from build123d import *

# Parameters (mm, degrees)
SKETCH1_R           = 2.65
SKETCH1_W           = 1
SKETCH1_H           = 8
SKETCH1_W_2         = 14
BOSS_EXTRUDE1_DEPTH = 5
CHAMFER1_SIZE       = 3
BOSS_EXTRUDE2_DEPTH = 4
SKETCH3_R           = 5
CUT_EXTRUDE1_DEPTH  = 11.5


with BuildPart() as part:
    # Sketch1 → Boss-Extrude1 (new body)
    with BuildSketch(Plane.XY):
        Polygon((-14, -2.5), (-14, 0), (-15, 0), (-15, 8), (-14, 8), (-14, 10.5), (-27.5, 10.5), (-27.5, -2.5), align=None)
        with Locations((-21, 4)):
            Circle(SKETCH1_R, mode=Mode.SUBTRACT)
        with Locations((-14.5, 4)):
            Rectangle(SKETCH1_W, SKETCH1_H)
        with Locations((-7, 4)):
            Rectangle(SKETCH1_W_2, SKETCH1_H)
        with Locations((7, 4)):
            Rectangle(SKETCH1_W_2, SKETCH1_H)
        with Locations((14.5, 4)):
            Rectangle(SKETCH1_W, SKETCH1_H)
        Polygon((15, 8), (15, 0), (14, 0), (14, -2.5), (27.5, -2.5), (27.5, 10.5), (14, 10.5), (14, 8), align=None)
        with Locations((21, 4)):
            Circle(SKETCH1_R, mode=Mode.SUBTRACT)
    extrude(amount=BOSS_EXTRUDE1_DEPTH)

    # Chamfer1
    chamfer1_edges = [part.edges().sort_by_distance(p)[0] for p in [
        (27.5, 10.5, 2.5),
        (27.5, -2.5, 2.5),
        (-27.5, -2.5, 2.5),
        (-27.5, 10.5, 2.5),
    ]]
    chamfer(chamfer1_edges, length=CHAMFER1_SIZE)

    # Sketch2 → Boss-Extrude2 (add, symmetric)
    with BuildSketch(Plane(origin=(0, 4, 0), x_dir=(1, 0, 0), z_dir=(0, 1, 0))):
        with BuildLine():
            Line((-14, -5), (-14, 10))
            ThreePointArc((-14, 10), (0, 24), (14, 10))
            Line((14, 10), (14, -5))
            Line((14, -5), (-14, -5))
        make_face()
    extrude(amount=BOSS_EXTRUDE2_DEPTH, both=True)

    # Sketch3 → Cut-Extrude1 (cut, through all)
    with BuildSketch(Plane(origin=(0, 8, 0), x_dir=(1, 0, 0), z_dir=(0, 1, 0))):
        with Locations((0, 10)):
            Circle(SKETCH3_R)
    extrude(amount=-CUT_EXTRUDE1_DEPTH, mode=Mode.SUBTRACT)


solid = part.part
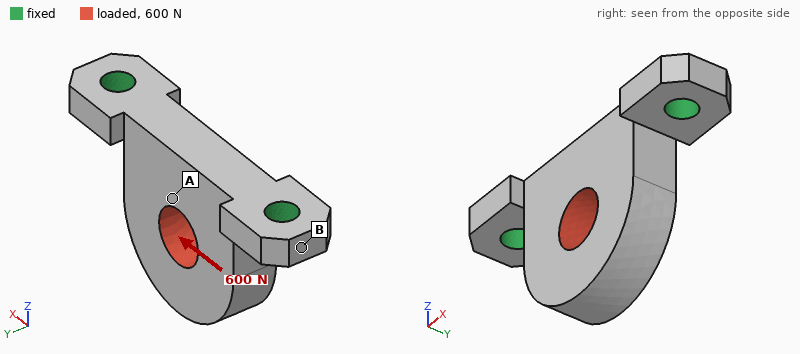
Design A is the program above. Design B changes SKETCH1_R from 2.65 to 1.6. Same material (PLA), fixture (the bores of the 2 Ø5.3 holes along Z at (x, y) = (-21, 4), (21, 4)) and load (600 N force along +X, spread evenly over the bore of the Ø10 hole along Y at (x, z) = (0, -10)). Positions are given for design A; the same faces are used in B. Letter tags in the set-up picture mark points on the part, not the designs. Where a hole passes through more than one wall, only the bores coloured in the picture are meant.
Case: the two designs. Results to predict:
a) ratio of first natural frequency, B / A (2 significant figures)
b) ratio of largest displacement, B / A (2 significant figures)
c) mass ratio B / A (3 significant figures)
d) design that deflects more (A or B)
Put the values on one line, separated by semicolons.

0.90; 1.2; 1.02; B
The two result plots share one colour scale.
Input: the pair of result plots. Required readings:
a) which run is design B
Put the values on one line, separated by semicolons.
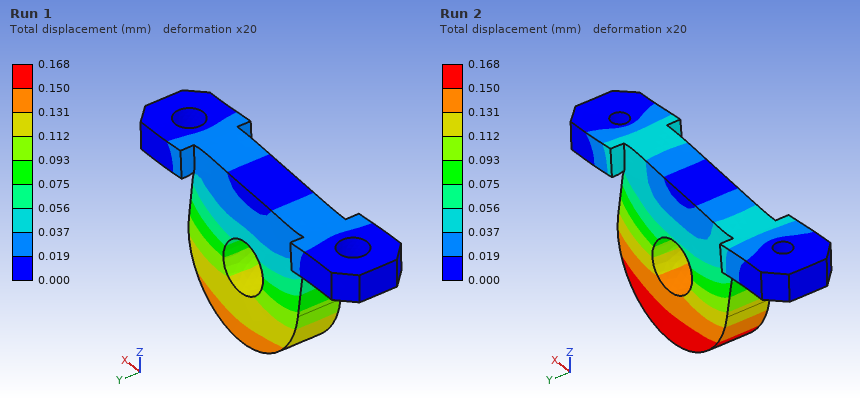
Run 2
